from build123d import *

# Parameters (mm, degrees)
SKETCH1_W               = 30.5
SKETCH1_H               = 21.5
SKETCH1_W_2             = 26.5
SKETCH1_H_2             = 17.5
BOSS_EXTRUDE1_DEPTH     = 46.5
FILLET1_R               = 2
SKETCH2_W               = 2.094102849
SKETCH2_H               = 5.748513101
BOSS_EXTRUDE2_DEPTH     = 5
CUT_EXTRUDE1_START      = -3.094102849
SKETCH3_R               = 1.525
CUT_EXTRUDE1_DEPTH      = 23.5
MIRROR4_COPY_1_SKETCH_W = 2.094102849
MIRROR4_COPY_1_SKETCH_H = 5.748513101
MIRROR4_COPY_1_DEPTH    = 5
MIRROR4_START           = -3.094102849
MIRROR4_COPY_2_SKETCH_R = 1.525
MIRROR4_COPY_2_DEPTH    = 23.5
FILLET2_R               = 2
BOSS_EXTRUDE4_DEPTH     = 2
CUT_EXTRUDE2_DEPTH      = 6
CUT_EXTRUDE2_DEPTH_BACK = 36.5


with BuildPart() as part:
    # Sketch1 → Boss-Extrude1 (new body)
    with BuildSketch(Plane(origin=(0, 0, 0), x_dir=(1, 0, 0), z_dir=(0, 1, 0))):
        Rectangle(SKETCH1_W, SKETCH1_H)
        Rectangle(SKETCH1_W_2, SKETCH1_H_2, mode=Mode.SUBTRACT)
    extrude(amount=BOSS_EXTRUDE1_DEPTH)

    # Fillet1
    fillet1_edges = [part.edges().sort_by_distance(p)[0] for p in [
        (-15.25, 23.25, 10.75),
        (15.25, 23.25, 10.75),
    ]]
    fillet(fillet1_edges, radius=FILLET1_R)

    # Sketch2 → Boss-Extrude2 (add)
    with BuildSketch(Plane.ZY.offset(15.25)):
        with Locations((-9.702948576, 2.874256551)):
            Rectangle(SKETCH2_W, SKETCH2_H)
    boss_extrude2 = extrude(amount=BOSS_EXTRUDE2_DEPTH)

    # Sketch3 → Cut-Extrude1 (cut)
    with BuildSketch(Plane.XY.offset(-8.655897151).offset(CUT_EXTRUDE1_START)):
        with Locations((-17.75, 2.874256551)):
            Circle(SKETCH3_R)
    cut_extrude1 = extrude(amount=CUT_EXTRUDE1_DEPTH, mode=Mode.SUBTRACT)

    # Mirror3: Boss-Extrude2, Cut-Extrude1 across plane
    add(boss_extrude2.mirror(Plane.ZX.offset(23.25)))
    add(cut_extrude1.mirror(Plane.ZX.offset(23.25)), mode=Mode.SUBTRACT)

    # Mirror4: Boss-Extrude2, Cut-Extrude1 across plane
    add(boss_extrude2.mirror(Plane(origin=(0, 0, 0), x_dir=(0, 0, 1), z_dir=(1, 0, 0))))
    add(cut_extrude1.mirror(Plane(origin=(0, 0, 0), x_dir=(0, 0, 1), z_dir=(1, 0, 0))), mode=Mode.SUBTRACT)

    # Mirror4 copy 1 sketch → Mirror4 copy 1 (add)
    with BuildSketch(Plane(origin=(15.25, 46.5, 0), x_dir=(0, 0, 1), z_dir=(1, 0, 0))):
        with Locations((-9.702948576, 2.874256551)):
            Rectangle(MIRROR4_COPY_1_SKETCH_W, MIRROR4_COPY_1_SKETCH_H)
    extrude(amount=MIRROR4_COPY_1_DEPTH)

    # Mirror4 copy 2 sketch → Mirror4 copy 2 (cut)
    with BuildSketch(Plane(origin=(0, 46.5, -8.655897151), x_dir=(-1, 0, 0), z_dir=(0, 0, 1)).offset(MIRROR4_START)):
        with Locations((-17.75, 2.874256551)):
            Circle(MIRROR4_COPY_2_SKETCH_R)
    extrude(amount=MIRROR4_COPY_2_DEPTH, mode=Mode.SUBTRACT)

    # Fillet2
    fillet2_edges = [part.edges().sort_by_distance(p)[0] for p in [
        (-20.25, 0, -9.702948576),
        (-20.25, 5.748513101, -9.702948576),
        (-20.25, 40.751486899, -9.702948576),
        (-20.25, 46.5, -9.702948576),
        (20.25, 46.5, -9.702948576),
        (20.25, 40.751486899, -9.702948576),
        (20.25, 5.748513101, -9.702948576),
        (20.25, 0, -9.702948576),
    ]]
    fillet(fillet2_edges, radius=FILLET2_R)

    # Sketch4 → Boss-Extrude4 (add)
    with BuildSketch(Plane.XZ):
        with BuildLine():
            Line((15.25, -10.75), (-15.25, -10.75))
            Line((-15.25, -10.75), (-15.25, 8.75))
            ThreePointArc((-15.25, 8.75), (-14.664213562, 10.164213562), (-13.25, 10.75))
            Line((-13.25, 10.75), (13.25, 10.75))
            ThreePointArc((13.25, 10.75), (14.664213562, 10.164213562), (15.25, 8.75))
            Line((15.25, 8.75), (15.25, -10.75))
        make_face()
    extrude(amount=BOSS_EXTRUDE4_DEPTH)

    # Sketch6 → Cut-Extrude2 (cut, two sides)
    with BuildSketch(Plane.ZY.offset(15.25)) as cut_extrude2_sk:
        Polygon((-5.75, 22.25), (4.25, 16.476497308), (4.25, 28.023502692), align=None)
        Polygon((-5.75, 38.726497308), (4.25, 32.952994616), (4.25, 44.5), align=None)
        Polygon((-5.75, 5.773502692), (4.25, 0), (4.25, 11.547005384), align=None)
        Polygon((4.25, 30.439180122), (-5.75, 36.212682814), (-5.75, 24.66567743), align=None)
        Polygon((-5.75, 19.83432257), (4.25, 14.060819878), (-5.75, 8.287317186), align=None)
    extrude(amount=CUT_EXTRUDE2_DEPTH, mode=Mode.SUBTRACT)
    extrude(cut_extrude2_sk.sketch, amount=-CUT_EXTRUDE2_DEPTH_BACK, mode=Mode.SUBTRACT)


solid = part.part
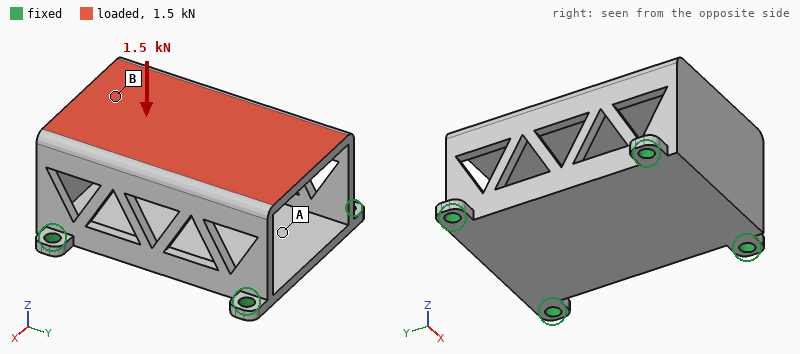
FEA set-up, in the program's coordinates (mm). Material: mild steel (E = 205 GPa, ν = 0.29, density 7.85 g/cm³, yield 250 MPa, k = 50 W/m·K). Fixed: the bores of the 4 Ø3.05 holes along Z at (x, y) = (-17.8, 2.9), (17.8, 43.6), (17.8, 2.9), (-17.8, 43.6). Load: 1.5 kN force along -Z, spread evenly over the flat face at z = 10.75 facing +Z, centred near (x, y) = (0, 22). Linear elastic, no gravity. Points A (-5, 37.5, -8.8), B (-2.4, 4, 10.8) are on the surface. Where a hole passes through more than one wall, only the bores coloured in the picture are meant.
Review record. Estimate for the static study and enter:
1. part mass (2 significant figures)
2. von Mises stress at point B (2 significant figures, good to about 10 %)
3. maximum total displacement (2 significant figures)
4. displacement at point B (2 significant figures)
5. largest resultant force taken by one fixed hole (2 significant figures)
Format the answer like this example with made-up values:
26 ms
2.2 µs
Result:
72 g
26 MPa
43 µm
12 µm
400 N
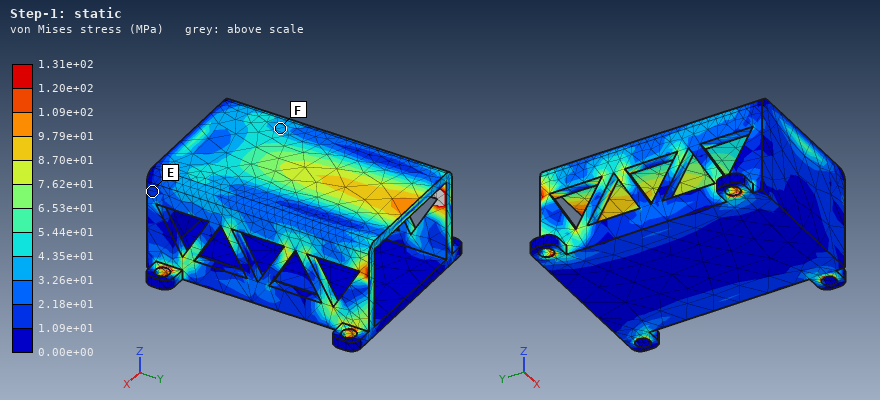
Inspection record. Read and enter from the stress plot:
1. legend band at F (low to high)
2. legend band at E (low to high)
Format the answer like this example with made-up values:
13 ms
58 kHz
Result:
3.26e+01 to 4.35e+01 MPa
1.09e+01 to 2.18e+01 MPa
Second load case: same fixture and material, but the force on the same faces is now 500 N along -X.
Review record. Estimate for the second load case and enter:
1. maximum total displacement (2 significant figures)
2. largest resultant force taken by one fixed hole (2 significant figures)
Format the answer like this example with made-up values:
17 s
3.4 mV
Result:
27 µm
420 N
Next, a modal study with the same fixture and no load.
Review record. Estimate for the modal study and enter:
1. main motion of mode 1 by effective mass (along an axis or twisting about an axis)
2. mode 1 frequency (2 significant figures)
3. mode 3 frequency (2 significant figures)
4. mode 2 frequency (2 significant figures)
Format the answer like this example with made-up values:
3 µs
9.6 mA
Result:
along X
4600 Hz
7600 Hz
7500 Hz
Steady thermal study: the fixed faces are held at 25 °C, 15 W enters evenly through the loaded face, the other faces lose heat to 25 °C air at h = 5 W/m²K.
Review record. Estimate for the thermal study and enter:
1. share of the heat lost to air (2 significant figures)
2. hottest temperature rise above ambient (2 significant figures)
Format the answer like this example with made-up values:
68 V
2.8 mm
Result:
11 %
79 K
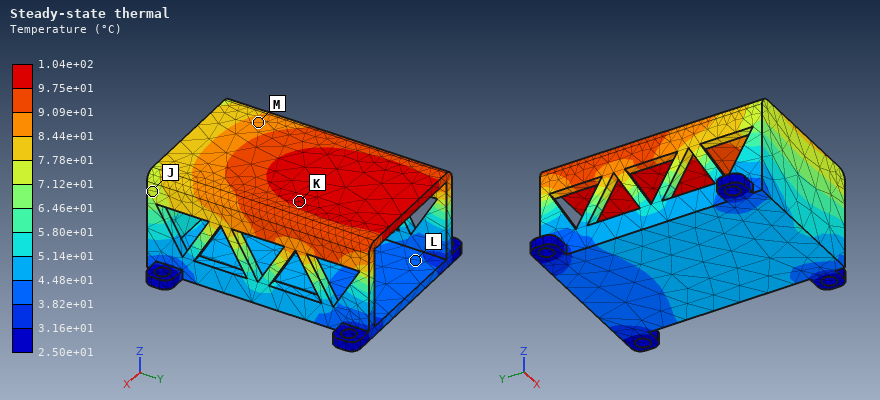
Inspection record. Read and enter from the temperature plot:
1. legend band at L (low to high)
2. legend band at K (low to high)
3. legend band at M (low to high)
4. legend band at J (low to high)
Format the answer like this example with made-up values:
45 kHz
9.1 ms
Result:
3.82e+01 to 4.48e+01 °C
9.75e+01 to 1.04e+02 °C
8.44e+01 to 9.09e+01 °C
7.12e+01 to 7.78e+01 °C
